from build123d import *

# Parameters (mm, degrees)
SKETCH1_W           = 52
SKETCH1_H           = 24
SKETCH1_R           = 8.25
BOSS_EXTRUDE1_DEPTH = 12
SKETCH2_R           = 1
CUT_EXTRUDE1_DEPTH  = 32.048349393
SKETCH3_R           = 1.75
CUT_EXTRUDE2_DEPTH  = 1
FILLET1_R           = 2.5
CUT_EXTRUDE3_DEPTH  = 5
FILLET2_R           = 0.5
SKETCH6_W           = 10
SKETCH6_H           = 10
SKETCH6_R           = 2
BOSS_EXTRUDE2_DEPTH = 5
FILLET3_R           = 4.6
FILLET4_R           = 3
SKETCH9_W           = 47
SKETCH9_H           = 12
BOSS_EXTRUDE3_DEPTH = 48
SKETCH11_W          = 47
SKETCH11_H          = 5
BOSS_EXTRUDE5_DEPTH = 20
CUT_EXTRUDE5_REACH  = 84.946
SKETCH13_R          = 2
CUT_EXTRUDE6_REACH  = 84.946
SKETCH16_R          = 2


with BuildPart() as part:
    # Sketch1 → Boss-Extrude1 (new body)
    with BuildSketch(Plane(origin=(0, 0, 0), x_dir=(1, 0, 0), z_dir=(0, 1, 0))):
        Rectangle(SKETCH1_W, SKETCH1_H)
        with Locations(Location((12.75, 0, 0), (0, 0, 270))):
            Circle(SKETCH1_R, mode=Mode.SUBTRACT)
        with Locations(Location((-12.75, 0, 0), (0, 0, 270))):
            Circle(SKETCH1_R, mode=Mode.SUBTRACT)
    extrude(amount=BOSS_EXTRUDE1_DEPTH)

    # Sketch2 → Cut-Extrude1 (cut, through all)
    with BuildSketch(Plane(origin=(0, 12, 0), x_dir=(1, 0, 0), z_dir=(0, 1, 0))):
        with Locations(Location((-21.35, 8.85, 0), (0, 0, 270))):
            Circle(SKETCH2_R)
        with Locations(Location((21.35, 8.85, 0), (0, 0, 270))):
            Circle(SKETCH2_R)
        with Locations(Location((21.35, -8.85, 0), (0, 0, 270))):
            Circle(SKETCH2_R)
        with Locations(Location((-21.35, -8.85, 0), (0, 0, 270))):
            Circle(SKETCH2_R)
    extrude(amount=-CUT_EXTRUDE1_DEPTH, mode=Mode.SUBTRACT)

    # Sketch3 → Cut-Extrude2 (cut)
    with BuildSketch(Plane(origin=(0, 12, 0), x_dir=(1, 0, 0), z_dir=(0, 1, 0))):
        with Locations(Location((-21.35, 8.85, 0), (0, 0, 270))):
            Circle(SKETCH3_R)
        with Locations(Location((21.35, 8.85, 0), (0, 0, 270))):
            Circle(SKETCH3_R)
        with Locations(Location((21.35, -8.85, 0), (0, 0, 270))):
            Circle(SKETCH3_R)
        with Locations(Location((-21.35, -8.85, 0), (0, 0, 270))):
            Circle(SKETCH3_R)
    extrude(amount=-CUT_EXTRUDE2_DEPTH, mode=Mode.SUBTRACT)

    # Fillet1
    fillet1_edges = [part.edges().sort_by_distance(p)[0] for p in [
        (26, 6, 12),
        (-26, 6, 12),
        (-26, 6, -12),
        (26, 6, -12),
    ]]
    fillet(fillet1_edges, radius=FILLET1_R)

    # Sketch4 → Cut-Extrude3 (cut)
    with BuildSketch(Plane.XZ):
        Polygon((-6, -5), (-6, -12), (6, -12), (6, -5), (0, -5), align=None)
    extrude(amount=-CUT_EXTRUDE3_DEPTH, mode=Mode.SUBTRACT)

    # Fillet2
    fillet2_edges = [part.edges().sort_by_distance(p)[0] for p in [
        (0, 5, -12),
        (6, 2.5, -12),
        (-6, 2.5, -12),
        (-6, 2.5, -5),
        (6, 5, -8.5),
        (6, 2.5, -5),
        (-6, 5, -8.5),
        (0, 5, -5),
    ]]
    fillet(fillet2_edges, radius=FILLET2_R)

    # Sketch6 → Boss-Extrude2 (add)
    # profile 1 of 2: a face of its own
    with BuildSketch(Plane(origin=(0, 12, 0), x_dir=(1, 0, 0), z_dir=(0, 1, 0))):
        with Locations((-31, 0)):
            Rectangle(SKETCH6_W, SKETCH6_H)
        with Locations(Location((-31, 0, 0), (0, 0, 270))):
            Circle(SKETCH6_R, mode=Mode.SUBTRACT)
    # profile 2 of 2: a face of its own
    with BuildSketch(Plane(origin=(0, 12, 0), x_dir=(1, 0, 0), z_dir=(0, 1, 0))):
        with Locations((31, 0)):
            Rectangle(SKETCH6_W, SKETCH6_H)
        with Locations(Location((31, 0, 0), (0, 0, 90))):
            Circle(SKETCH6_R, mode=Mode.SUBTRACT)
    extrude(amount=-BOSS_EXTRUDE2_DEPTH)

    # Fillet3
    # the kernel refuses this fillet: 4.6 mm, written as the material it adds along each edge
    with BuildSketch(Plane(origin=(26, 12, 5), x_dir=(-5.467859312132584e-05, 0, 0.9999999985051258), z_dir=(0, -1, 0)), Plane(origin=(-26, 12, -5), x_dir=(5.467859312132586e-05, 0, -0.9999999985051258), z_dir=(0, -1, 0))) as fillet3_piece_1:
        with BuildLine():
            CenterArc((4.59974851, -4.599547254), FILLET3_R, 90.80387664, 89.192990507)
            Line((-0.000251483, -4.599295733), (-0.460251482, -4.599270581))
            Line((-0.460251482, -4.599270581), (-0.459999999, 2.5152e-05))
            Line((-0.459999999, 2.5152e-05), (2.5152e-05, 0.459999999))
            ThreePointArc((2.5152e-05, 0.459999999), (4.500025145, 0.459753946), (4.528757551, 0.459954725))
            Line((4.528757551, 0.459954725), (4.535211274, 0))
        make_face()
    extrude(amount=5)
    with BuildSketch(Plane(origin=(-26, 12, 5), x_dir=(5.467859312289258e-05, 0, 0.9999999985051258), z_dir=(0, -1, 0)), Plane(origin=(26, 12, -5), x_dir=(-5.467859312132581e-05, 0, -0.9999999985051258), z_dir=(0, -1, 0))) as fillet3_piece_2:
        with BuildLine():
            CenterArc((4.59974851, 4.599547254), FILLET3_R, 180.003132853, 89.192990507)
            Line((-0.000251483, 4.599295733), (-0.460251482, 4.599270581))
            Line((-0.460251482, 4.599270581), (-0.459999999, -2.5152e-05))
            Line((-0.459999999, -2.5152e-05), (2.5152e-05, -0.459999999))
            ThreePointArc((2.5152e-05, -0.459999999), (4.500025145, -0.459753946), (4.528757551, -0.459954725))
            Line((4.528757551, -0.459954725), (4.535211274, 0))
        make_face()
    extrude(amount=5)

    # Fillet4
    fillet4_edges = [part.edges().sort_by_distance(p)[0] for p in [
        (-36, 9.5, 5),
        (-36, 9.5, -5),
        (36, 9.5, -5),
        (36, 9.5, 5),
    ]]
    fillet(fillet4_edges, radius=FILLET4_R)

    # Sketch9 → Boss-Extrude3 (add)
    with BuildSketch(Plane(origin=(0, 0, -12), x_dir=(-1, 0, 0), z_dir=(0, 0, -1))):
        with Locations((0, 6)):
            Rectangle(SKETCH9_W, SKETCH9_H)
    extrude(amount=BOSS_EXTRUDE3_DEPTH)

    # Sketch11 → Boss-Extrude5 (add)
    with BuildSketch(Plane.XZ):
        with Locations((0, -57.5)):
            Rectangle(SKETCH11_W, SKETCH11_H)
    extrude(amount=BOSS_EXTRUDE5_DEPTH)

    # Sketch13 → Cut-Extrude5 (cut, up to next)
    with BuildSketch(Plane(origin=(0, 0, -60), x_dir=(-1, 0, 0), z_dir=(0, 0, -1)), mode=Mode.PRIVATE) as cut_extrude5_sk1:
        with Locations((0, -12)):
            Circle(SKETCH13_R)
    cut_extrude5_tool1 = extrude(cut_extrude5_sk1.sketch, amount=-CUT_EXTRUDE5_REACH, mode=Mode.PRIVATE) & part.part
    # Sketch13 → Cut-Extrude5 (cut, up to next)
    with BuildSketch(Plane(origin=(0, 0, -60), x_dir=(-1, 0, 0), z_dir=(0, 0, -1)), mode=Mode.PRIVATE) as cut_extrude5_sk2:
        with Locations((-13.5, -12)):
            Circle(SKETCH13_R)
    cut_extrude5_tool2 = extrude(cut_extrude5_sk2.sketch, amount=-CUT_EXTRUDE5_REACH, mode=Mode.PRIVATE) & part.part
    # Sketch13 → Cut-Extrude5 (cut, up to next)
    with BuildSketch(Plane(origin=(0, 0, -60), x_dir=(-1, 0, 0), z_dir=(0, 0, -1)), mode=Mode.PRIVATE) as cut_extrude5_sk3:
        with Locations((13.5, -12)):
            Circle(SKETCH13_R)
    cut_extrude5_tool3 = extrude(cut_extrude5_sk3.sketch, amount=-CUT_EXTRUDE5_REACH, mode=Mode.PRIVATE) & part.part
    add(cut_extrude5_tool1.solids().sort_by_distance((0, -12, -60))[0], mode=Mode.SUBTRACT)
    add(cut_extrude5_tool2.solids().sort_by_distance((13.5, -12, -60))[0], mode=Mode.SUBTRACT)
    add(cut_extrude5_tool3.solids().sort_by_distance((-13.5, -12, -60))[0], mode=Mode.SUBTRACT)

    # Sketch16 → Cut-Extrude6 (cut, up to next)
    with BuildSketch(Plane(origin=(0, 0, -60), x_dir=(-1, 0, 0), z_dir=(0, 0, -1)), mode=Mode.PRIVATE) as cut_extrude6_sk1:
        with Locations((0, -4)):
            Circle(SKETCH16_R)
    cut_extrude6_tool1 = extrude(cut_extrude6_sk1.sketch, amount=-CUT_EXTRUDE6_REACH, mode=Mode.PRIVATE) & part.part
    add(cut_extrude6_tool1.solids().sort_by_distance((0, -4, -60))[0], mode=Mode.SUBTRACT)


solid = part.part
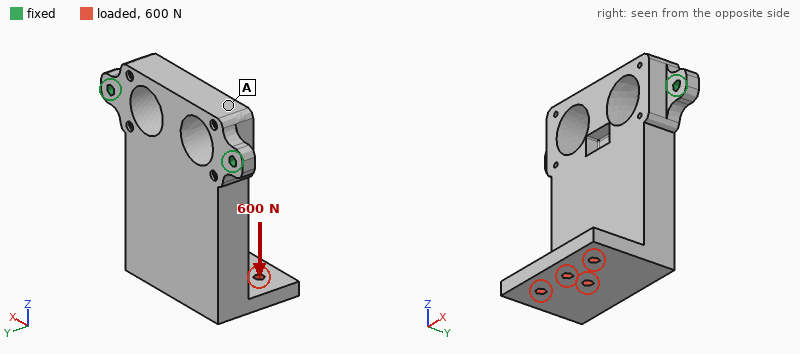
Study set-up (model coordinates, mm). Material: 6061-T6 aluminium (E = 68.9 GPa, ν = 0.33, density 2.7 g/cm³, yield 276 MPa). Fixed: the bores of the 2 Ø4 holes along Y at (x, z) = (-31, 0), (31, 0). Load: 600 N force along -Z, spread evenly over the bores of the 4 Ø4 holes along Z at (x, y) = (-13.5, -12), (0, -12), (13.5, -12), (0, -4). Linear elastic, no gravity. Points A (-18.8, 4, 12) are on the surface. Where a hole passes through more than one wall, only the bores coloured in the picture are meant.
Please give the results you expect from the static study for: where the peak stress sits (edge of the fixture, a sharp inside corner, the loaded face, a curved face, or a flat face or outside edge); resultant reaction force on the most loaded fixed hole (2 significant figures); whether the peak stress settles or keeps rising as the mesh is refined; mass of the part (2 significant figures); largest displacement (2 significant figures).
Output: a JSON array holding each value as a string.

["edge of the fixture", "300 N", "keeps rising", "110 g", "0.30 mm"]
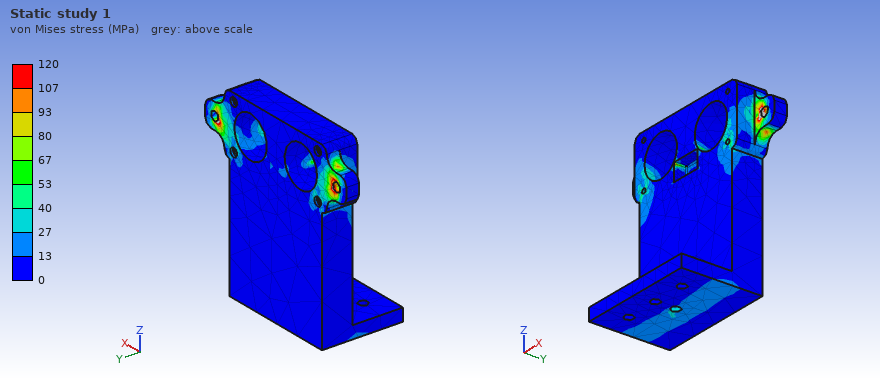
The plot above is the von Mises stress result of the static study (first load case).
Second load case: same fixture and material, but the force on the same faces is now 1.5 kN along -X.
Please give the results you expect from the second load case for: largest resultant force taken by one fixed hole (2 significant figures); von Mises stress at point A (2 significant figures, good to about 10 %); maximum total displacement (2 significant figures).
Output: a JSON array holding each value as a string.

["1.7 kN", "6.9 MPa", "0.11 mm"]
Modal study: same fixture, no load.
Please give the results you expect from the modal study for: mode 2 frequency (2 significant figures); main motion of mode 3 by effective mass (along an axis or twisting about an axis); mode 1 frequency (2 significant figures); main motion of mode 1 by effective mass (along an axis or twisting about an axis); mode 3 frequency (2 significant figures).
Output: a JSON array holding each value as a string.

["4200 Hz", "along X", "700 Hz", "along Y", "4800 Hz"]
